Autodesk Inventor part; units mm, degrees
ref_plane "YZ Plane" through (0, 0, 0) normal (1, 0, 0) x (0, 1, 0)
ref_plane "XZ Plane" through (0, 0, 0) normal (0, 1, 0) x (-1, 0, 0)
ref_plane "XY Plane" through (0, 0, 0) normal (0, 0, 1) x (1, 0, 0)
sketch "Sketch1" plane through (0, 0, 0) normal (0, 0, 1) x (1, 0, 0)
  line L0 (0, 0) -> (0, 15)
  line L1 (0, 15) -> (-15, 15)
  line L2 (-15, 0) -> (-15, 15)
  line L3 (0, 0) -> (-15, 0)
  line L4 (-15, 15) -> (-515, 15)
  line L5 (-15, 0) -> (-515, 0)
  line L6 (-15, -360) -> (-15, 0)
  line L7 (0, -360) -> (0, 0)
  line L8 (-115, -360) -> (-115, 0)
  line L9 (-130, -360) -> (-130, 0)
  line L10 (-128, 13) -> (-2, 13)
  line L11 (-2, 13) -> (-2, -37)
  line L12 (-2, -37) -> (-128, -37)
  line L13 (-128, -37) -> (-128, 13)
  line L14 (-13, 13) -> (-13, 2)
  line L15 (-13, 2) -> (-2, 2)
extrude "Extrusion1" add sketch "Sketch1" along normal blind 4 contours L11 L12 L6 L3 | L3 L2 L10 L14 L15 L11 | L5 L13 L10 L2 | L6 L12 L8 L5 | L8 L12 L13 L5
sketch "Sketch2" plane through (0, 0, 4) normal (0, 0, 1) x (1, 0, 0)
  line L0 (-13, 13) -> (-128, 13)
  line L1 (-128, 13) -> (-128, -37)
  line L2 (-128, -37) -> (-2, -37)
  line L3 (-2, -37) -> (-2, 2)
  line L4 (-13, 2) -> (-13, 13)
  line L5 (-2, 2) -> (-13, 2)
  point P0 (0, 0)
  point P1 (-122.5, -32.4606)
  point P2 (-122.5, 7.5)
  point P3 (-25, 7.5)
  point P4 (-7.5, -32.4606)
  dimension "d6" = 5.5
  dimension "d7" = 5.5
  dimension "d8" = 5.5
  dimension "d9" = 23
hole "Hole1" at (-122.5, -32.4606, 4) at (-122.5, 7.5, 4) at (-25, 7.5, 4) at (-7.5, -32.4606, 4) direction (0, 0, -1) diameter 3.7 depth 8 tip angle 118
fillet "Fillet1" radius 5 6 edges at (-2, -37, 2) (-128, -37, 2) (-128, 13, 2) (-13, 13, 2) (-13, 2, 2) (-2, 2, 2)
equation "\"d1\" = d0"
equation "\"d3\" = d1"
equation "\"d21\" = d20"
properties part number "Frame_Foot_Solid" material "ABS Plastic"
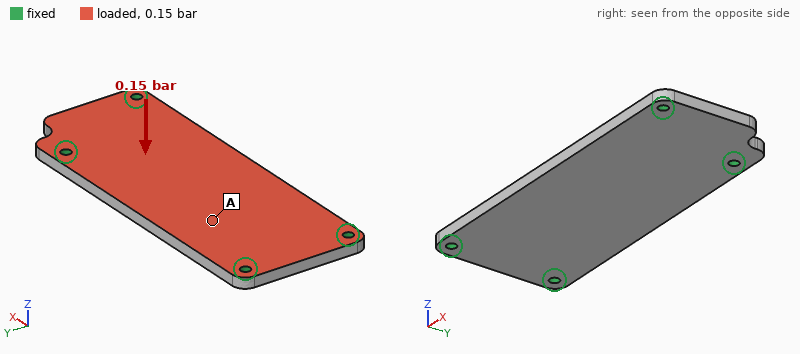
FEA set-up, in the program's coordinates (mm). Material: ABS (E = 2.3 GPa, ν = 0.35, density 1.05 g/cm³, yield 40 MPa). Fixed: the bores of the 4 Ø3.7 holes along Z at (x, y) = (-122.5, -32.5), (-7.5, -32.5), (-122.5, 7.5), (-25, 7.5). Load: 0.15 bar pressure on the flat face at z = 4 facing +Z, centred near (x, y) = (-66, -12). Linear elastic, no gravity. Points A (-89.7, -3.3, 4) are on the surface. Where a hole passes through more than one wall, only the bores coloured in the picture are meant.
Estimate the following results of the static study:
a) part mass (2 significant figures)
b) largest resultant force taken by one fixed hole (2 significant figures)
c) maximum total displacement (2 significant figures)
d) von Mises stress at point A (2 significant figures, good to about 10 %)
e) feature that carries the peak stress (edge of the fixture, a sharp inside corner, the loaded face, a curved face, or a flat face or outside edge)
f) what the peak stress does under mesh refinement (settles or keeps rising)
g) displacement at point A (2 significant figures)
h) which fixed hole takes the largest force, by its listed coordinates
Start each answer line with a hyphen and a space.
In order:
- 26 g
- 33 N
- 0.56 mm
- 1.6 MPa
- edge of the fixture
- keeps rising
- 0.32 mm
- (-25, 7.5)
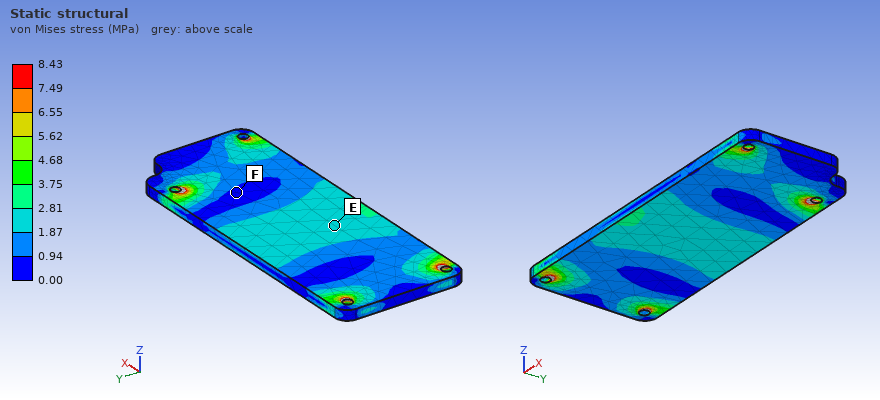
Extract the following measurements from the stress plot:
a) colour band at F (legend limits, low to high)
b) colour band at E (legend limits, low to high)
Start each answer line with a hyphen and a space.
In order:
- 0.00 to 0.94 MPa
- 1.87 to 2.81 MPa
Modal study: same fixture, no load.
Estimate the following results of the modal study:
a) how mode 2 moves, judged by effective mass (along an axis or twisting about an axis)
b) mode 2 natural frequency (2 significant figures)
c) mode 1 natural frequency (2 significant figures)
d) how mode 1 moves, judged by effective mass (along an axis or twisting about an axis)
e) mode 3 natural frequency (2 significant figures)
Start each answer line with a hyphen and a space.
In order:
- twisting about X
- 910 Hz
- 510 Hz
- along Z
- 1400 Hz
